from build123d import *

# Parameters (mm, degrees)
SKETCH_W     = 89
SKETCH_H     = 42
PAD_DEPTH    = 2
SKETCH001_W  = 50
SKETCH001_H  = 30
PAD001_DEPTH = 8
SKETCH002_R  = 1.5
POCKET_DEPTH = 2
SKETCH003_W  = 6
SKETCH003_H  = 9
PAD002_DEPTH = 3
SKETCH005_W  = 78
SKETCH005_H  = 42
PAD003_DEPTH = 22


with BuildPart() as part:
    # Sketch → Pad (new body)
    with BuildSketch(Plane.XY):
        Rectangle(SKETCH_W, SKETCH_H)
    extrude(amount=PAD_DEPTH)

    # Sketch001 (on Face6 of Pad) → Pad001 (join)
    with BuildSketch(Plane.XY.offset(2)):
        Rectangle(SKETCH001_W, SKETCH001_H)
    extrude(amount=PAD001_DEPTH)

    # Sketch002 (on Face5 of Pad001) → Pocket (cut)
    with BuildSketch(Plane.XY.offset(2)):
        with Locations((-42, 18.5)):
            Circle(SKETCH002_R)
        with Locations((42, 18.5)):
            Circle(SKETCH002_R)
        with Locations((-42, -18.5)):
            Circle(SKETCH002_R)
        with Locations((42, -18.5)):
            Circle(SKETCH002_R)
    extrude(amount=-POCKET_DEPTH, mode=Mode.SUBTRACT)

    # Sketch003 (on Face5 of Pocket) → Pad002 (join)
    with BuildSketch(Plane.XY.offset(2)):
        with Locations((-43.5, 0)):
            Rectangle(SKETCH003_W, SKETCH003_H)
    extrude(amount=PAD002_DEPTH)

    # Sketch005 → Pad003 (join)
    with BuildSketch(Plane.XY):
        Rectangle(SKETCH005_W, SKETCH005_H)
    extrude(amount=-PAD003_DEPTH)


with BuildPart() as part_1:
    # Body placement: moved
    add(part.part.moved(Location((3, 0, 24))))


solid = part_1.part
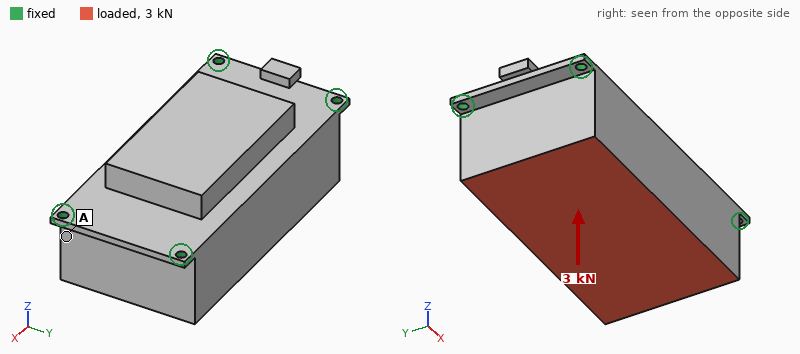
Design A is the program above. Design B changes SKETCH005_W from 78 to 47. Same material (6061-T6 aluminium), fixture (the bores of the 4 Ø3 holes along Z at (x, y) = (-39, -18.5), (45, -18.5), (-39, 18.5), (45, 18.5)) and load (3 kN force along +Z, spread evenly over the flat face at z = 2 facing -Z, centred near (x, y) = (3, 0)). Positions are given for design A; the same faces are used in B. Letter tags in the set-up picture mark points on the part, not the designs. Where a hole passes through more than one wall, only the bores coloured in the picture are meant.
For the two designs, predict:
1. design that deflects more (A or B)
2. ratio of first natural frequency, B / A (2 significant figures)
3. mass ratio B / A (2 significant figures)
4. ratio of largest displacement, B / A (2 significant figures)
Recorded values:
B
0.21
0.69
32
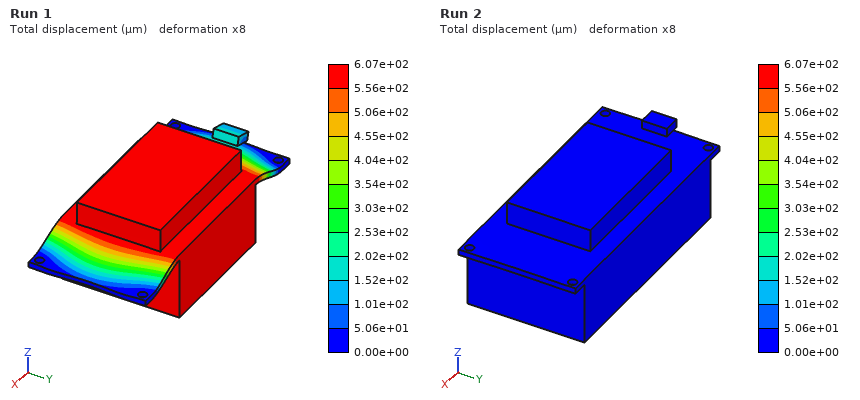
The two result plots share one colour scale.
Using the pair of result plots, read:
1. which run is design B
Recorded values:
Run 1
